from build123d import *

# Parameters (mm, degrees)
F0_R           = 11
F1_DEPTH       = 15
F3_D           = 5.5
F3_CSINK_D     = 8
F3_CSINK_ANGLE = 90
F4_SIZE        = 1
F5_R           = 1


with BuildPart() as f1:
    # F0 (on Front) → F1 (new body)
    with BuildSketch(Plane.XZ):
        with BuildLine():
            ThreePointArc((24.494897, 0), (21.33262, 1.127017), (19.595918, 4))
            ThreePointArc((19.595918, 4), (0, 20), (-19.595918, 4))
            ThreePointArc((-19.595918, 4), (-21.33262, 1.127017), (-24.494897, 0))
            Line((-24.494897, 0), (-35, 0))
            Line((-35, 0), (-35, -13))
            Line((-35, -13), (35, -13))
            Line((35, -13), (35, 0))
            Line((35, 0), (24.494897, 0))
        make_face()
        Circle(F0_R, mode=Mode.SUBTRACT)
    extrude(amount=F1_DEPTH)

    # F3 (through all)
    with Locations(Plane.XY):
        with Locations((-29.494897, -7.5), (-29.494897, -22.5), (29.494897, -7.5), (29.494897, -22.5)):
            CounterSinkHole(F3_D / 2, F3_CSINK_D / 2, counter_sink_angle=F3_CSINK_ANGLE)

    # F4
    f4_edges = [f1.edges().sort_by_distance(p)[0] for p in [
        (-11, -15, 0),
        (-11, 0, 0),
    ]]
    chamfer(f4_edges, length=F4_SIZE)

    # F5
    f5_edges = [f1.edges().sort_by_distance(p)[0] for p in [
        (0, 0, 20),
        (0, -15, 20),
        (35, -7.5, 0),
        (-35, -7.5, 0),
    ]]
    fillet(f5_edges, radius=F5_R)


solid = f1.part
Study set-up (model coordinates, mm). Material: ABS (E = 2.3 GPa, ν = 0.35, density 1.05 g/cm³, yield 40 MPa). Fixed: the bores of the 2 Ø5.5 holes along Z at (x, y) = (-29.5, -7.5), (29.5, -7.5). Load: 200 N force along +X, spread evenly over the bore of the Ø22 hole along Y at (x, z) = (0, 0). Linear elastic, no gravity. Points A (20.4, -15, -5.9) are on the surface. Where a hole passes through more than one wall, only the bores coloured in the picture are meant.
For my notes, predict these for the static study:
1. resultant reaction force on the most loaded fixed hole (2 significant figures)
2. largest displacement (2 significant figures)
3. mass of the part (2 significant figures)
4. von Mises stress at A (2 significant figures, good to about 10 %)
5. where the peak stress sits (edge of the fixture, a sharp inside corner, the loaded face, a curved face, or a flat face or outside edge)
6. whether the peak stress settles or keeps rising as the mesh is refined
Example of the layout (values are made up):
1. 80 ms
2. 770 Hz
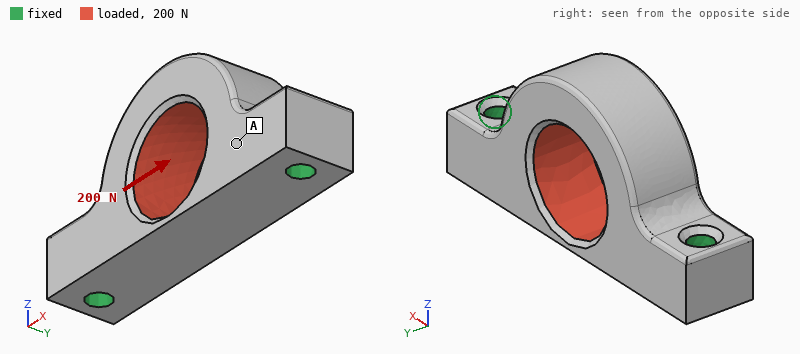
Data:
1. 100 N
2. 14 µm
3. 18 g
4. 0.26 MPa
5. edge of the fixture
6. keeps rising
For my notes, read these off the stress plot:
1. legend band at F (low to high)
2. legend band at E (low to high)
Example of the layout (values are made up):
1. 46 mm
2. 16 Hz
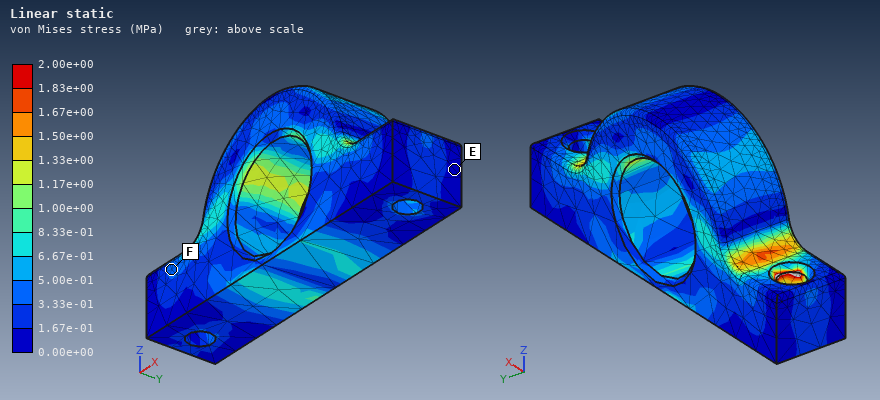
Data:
1. 3.33e-01 to 5.00e-01 MPa
2. 0.00e+00 to 1.67e-01 MPa
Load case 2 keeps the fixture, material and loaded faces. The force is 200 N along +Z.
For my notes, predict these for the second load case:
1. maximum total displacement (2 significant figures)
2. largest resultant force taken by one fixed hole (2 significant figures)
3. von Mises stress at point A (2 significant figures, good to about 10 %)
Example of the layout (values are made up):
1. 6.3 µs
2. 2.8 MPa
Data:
1. 32 µm
2. 100 N
3. 1.0 MPa
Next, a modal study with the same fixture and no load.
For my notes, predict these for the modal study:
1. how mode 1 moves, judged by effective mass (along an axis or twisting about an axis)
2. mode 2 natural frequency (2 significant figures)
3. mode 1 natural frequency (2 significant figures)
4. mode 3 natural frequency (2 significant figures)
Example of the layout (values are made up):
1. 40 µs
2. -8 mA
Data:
1. along Y
2. 5100 Hz
3. 2300 Hz
4. 5200 Hz
